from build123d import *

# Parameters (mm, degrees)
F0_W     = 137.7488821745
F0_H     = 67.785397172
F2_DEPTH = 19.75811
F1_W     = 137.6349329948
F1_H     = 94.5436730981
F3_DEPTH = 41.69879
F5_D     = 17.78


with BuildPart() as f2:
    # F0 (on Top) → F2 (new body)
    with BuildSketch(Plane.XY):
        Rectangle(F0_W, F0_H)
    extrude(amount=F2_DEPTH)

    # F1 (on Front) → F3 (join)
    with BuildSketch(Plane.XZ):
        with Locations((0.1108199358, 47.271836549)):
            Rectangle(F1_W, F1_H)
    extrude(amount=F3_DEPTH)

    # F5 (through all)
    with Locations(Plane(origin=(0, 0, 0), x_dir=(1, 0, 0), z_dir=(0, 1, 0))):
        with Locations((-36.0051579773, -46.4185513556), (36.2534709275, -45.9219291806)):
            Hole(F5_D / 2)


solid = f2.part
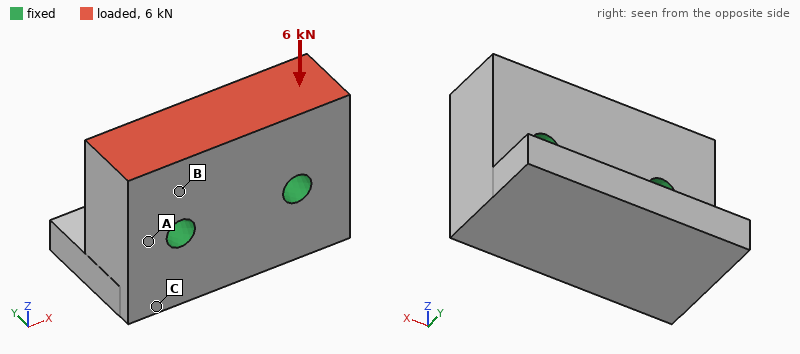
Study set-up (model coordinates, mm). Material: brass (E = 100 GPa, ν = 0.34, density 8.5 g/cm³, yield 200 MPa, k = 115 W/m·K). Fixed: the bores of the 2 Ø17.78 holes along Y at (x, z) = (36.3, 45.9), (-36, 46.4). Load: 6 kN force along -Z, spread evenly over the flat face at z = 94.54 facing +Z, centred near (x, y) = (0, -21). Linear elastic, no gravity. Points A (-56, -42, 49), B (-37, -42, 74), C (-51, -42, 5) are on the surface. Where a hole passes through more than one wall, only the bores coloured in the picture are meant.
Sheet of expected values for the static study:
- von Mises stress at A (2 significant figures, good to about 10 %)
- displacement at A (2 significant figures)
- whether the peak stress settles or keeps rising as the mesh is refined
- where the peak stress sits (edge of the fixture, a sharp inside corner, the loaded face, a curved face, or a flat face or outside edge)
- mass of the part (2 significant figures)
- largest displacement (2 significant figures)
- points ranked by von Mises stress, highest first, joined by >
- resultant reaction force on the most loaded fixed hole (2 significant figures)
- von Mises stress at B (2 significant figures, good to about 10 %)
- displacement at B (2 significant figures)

0.65 MPa
0.24 µm
keeps rising
edge of the fixture
5.2 kg
0.78 µm
B > A > C
3.0 kN
1.3 MPa
0.33 µm
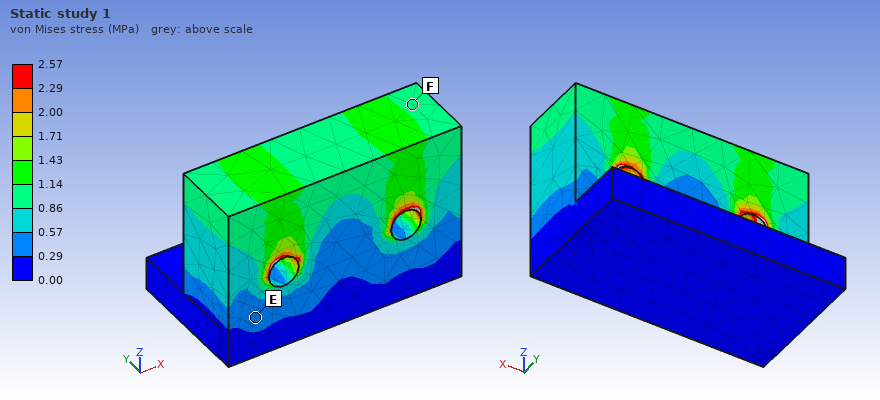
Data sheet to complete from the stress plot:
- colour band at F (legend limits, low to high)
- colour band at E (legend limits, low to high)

0.86 to 1.14 MPa
0.29 to 0.57 MPa
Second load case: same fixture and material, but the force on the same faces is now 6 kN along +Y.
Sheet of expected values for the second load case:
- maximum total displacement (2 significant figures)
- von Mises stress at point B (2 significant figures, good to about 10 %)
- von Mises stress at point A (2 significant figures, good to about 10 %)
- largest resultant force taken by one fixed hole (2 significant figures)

5.2 µm
3.7 MPa
3.1 MPa
3.0 kN
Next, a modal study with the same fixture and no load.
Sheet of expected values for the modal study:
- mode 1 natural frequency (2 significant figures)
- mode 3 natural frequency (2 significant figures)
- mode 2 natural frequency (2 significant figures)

3900 Hz
5800 Hz
4800 Hz
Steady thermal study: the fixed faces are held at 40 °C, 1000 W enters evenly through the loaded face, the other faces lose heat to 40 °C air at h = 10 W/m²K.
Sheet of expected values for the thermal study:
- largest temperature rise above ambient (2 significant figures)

75 K
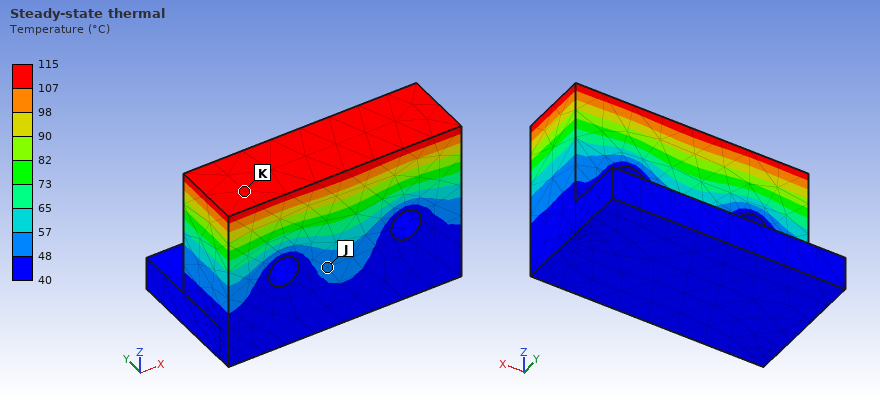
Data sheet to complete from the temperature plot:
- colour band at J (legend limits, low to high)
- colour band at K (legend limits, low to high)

48 to 57 °C
107 to 115 °C
